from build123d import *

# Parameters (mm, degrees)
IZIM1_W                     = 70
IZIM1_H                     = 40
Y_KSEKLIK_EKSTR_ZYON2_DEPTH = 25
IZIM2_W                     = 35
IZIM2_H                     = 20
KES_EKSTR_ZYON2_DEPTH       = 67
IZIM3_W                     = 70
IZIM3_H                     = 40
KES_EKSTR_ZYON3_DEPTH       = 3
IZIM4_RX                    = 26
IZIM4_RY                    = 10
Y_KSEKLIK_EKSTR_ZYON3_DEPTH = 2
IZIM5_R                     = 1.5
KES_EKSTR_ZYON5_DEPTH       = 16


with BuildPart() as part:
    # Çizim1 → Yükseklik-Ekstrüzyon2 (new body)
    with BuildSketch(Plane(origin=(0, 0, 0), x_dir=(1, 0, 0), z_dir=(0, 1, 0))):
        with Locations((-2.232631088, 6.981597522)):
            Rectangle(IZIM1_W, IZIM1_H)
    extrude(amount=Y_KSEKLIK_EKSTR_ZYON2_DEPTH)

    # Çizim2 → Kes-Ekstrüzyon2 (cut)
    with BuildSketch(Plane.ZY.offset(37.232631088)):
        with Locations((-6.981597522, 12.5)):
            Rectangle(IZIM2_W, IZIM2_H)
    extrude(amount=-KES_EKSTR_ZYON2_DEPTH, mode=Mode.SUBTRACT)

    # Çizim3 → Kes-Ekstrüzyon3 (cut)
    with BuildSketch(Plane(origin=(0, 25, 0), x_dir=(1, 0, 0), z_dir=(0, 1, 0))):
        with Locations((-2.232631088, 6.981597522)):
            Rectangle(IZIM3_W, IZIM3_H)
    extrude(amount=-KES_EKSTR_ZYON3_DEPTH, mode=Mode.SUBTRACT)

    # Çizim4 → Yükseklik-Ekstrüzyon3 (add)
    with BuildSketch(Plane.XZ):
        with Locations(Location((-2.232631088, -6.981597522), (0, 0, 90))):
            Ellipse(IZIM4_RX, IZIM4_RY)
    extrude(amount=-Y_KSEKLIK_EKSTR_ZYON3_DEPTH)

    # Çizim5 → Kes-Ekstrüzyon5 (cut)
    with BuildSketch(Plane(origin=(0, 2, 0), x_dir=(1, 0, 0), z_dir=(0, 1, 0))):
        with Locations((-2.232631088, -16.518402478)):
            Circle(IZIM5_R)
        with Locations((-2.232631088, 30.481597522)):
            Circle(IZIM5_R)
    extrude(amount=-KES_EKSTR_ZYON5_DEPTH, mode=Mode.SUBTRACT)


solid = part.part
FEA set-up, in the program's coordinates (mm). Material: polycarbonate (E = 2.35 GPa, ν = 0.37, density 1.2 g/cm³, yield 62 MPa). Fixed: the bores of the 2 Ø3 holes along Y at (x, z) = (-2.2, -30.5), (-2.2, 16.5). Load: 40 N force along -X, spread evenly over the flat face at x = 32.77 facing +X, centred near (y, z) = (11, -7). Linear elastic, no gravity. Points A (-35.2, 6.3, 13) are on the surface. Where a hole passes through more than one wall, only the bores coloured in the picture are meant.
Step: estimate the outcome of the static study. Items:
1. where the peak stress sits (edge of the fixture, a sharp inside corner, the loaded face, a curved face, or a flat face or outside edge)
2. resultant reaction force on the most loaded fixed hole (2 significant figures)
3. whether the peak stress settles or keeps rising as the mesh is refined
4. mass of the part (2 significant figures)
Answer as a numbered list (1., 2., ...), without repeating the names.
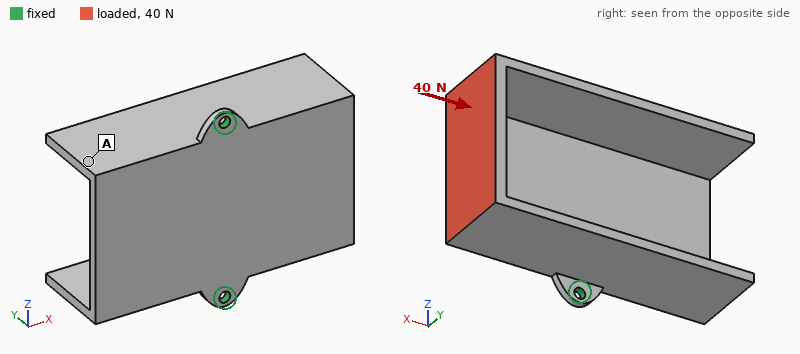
1. edge of the fixture
2. 20 N
3. keeps rising
4. 19 g
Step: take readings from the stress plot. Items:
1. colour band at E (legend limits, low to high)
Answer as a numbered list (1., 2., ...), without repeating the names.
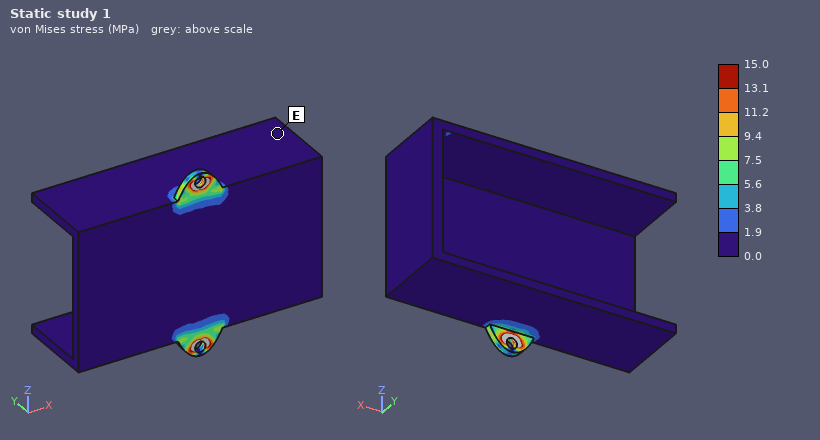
1. 0.0 to 1.9 MPa
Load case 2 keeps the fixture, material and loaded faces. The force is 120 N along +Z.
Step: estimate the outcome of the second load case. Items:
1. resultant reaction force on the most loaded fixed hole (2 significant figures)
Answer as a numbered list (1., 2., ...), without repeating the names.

1. 110 N
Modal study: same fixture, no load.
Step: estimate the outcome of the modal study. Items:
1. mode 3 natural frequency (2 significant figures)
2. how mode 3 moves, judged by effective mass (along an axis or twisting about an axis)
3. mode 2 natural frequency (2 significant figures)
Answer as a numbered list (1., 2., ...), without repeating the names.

1. 730 Hz
2. along Y
3. 580 Hz
